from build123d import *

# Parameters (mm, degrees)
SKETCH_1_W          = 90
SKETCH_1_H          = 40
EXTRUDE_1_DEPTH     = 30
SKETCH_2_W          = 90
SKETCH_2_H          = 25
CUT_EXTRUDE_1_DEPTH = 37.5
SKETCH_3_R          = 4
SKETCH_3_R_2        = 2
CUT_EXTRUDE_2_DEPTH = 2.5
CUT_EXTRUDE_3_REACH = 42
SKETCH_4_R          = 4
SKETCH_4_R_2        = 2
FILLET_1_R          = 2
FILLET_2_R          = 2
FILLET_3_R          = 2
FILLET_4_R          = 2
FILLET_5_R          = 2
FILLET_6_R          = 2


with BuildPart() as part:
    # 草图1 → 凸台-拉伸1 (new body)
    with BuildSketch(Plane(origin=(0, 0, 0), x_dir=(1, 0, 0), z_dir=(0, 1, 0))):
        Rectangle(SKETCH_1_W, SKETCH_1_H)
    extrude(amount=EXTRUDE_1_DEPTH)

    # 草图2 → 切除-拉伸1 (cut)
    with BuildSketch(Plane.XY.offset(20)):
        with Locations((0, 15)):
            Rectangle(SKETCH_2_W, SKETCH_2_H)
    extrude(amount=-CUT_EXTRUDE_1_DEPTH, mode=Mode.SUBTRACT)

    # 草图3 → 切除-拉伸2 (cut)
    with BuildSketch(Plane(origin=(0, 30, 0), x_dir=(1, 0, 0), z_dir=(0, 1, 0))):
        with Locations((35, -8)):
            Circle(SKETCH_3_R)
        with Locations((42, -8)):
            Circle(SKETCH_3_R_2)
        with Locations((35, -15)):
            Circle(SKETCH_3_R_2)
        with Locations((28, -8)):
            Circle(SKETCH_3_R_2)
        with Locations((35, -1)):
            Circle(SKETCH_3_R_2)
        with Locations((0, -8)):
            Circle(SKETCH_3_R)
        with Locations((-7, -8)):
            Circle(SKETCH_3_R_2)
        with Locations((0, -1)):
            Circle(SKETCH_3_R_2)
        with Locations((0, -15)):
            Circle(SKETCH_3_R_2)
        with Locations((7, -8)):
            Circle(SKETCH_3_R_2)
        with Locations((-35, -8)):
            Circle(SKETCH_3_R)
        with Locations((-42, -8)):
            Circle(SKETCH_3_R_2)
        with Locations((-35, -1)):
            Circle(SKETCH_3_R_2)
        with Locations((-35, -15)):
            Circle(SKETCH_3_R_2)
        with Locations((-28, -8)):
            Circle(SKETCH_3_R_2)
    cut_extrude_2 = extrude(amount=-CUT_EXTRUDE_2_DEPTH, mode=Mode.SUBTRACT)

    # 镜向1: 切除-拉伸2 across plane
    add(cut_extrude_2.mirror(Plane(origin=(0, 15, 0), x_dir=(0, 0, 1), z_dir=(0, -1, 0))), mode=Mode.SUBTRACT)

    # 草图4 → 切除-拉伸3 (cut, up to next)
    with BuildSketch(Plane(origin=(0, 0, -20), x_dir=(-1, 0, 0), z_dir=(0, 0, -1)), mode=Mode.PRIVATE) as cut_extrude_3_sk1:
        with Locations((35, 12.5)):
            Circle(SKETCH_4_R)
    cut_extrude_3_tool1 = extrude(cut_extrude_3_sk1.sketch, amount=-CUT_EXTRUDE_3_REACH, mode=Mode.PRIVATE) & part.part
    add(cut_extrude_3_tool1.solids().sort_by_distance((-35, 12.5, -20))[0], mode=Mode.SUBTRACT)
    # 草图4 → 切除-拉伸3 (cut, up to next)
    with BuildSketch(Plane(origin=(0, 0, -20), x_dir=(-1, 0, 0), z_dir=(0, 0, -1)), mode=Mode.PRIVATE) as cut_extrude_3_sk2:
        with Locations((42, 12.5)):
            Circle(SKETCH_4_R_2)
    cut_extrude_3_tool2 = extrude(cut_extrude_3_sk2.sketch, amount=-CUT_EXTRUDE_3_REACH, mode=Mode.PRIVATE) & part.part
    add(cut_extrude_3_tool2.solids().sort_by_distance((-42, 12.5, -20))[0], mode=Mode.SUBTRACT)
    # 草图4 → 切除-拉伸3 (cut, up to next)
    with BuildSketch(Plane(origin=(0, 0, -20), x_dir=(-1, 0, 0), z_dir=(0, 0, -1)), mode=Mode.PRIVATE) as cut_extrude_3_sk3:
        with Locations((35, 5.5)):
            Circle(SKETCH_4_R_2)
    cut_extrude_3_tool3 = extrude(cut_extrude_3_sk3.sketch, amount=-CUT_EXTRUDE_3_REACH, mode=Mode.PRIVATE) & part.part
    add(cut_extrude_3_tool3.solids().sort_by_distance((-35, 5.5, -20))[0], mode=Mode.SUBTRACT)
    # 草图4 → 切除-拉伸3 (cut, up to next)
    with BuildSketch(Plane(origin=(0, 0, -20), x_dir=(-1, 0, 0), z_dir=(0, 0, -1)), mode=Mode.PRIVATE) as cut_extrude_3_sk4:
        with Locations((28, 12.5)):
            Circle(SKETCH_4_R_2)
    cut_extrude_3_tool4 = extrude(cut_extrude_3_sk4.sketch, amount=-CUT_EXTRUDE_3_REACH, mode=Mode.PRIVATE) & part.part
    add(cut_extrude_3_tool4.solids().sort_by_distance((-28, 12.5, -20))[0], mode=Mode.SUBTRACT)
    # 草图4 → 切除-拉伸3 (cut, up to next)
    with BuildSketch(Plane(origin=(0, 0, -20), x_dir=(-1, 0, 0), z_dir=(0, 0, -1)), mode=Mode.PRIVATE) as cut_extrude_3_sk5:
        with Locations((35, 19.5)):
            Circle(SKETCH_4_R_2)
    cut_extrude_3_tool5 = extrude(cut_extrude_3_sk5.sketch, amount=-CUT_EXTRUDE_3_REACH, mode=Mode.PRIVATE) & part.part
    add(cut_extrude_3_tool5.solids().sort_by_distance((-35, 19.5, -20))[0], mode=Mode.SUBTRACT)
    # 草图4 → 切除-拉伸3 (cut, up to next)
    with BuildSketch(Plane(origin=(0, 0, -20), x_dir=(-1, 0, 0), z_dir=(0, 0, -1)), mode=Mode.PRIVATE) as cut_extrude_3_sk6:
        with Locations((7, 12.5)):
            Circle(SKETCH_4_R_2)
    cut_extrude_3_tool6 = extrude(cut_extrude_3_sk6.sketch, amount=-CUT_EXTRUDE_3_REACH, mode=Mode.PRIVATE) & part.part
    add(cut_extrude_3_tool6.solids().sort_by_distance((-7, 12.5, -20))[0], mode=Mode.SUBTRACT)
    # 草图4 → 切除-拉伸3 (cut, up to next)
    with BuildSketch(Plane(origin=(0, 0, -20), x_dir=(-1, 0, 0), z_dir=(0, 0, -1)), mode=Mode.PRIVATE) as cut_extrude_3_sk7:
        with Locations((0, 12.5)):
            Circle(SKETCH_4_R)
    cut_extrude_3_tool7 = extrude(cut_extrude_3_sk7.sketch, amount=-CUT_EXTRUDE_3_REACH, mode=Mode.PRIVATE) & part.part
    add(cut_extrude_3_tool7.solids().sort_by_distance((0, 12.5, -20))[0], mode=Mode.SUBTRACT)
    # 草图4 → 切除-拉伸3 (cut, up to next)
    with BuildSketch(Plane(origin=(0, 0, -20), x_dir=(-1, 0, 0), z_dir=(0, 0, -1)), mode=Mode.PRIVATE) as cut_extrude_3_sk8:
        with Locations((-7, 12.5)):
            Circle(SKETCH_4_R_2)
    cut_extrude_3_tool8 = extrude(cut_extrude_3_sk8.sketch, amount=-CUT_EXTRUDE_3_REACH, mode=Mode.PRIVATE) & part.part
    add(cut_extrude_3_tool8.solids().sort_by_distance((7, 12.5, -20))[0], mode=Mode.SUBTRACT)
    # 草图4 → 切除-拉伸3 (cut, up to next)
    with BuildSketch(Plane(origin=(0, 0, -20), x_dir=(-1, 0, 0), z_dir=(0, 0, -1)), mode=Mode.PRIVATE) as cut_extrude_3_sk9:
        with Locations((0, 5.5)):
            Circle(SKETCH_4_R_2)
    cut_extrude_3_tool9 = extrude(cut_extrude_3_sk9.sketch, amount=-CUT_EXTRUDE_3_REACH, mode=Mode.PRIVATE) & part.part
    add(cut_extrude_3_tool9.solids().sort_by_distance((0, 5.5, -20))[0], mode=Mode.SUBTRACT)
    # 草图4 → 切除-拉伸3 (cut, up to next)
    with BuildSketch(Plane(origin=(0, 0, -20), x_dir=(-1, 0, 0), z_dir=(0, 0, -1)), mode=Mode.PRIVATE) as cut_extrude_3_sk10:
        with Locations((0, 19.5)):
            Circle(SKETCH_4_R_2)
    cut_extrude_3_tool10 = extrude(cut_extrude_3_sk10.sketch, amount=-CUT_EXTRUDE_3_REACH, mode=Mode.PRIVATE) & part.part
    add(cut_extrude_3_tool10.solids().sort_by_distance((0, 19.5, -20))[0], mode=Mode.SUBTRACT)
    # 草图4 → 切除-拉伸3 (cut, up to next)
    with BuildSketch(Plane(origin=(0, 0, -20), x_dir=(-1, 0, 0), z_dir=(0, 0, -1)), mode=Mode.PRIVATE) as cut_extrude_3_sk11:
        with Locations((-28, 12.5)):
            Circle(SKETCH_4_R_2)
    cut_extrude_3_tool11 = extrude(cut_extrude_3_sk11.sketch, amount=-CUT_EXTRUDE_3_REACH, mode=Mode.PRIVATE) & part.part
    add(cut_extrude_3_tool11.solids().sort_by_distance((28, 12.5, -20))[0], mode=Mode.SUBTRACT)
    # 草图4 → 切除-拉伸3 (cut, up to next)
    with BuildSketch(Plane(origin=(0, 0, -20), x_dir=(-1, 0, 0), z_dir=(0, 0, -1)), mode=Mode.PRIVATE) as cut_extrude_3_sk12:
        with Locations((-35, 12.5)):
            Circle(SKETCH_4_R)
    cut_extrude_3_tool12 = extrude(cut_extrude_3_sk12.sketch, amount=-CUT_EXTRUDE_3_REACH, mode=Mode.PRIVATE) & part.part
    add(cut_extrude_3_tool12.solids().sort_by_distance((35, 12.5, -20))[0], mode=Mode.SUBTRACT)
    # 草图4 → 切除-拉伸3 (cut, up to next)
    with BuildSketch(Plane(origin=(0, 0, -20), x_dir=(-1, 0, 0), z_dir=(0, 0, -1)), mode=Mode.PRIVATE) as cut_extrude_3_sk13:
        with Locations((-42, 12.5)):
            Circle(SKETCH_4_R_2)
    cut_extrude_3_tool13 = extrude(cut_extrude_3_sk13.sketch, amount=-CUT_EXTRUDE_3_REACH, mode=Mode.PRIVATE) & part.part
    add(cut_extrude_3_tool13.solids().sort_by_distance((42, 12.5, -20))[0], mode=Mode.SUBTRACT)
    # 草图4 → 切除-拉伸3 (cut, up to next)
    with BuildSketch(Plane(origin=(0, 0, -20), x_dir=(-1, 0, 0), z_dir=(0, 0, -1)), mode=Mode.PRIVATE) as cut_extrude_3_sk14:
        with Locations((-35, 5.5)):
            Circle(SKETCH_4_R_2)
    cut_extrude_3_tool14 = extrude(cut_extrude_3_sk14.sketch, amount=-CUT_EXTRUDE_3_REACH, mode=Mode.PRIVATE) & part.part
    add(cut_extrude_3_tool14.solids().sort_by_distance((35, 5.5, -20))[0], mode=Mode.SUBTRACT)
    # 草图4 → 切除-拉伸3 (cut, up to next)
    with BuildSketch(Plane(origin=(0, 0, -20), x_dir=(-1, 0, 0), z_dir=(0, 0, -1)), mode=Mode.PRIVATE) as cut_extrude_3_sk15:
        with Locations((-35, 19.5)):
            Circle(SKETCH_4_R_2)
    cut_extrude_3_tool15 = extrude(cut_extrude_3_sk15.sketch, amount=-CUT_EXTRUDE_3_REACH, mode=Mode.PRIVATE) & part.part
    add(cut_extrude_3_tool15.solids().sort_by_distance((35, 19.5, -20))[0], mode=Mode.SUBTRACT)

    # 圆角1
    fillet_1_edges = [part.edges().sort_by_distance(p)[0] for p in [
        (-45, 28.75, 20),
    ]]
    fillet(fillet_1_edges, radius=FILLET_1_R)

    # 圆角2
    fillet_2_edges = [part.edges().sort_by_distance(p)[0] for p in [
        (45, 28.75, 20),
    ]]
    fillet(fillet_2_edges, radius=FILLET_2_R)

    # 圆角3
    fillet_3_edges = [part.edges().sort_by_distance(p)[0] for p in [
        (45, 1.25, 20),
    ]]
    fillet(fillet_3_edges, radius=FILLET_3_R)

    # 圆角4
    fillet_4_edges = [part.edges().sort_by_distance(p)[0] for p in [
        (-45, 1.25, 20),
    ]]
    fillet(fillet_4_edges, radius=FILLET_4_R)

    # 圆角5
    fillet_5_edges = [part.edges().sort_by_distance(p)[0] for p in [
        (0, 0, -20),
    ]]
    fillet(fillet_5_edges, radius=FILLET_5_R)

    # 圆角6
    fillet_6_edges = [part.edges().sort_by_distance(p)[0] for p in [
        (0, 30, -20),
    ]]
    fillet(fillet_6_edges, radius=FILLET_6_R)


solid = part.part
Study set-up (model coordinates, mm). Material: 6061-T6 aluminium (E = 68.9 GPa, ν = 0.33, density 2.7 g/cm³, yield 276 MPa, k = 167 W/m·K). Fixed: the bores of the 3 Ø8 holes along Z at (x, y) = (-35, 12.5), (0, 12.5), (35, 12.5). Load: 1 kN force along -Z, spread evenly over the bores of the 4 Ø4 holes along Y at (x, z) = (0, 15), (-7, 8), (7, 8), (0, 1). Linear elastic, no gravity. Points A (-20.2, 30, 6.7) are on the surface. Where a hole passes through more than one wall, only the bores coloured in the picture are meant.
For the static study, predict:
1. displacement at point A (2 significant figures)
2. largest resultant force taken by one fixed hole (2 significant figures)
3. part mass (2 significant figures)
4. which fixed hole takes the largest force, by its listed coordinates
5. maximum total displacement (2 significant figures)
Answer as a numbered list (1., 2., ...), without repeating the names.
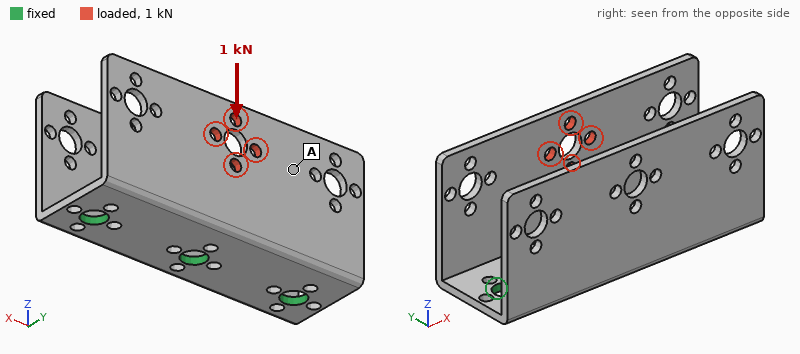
1. 0.43 mm
2. 430 N
3. 57 g
4. (0, 12.5)
5. 0.62 mm
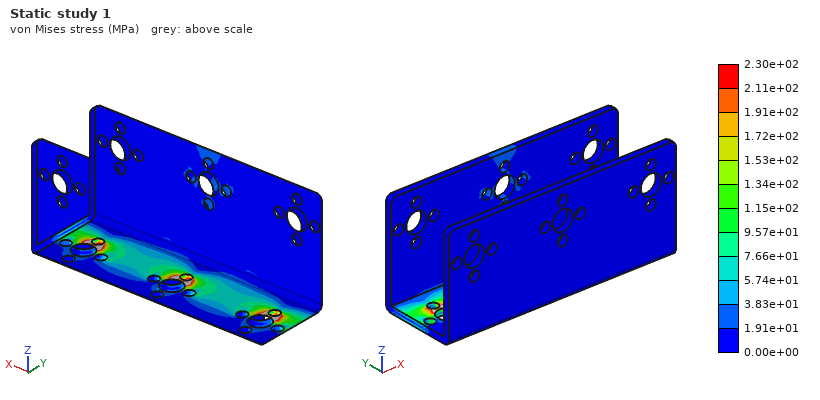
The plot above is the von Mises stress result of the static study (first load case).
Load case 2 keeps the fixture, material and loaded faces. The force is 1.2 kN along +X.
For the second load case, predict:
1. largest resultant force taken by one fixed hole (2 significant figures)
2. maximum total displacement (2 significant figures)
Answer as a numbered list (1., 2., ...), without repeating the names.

1. 620 N
2. 0.44 mm
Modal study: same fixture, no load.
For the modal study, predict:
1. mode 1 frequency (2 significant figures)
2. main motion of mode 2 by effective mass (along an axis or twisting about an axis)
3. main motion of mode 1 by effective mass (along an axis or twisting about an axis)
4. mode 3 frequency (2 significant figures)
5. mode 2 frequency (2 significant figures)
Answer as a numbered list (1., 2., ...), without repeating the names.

1. 900 Hz
2. along Y
3. along Y
4. 1500 Hz
5. 1000 Hz
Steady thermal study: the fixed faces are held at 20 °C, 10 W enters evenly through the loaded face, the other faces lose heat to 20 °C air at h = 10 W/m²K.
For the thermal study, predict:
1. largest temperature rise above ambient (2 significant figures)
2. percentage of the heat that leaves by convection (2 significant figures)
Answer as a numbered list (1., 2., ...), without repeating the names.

1. 18 K
2. 8.0 %
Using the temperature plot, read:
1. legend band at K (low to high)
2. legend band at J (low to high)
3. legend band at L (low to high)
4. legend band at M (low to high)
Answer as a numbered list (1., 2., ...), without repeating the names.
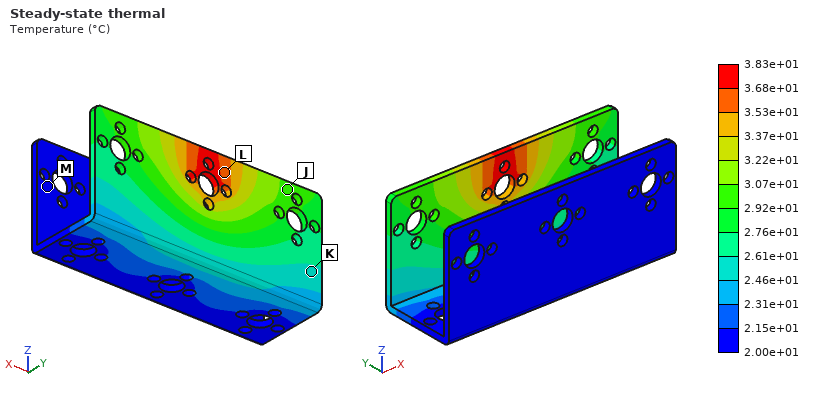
1. 2.46e+01 to 2.61e+01 °C
2. 2.92e+01 to 3.07e+01 °C
3. 3.53e+01 to 3.68e+01 °C
4. 2.00e+01 to 2.15e+01 °C
